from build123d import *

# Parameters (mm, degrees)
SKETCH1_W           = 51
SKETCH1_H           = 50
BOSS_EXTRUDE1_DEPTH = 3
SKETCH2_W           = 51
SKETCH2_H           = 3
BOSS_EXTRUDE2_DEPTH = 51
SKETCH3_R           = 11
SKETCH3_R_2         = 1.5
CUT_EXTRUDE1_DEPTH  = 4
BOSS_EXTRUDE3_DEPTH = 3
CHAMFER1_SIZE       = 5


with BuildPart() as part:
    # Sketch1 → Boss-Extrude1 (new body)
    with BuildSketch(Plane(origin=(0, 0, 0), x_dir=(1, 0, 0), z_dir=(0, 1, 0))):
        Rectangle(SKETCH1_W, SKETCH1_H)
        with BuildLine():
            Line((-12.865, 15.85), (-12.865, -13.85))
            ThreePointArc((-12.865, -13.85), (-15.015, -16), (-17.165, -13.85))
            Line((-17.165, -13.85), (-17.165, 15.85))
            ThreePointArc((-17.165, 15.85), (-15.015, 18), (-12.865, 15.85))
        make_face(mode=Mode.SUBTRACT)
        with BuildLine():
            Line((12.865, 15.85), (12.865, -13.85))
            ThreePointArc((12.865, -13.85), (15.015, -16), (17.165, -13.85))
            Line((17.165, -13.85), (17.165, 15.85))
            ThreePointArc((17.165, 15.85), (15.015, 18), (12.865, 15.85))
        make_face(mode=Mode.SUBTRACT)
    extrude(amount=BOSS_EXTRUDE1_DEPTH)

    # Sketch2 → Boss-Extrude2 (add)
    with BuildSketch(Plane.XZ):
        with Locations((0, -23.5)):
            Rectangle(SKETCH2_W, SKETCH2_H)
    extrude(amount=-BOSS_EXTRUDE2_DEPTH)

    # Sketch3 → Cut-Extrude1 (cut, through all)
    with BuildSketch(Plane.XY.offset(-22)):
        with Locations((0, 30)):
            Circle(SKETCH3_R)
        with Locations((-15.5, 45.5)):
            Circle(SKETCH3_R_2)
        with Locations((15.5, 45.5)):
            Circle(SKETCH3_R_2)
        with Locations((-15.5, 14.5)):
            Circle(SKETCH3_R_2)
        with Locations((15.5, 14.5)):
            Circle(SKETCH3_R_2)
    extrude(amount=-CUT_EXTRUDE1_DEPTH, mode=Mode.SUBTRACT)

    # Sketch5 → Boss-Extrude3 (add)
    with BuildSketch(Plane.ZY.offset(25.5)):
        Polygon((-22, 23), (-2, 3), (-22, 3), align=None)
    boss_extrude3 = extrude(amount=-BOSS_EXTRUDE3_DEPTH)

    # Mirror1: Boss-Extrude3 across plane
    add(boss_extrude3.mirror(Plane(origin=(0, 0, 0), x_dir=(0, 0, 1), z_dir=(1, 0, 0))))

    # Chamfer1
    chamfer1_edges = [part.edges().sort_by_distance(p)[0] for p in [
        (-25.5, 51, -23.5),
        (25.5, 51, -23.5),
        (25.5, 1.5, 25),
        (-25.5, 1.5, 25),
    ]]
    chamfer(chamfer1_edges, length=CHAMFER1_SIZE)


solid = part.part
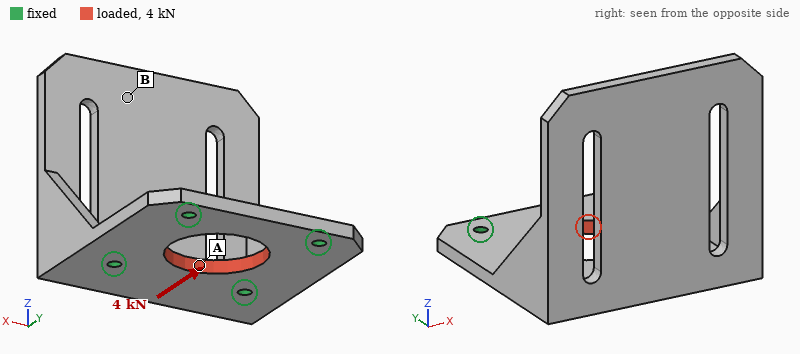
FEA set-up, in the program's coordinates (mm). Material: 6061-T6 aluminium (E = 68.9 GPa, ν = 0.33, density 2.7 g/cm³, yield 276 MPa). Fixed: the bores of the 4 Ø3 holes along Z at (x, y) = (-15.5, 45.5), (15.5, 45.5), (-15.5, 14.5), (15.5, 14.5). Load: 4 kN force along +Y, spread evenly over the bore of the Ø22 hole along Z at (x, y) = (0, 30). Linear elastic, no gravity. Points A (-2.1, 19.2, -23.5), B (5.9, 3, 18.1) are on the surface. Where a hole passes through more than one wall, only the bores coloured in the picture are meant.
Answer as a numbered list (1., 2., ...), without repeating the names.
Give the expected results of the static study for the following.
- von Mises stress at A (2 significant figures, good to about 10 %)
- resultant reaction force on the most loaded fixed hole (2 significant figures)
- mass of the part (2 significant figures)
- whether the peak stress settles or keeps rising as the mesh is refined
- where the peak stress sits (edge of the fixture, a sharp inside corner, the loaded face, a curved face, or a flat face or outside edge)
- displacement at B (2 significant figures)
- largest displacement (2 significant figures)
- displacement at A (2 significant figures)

1. 19 MPa
2. 1.0 kN
3. 38 g
4. keeps rising
5. edge of the fixture
6. 4.6 µm
7. 12 µm
8. 7.1 µm
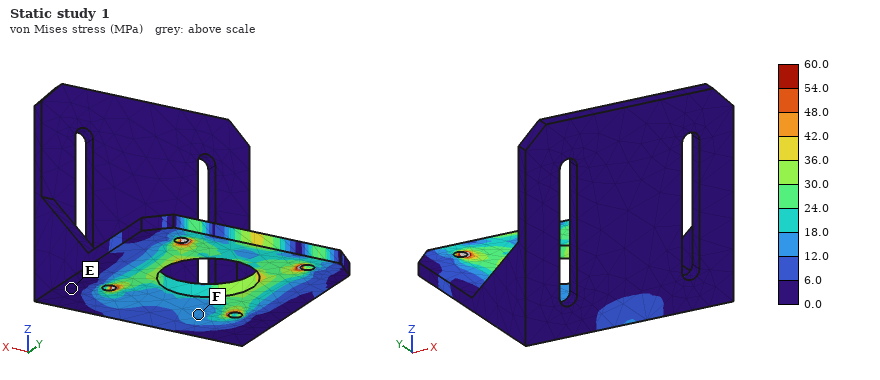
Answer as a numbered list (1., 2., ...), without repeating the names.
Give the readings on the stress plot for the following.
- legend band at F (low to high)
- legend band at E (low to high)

1. 12.0 to 18.0 MPa
2. 0.0 to 6.0 MPa
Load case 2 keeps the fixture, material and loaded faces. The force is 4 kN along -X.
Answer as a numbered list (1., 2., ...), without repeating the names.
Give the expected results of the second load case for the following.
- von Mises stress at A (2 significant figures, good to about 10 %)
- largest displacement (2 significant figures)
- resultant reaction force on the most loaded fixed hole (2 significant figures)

1. 33 MPa
2. 9.3 µm
3. 1.0 kN
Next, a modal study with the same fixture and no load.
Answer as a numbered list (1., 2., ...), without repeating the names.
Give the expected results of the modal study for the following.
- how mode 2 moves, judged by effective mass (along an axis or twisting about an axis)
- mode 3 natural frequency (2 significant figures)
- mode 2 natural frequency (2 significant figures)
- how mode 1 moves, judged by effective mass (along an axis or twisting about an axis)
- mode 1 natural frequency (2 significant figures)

1. along X
2. 4100 Hz
3. 2300 Hz
4. along Y
5. 1200 Hz
